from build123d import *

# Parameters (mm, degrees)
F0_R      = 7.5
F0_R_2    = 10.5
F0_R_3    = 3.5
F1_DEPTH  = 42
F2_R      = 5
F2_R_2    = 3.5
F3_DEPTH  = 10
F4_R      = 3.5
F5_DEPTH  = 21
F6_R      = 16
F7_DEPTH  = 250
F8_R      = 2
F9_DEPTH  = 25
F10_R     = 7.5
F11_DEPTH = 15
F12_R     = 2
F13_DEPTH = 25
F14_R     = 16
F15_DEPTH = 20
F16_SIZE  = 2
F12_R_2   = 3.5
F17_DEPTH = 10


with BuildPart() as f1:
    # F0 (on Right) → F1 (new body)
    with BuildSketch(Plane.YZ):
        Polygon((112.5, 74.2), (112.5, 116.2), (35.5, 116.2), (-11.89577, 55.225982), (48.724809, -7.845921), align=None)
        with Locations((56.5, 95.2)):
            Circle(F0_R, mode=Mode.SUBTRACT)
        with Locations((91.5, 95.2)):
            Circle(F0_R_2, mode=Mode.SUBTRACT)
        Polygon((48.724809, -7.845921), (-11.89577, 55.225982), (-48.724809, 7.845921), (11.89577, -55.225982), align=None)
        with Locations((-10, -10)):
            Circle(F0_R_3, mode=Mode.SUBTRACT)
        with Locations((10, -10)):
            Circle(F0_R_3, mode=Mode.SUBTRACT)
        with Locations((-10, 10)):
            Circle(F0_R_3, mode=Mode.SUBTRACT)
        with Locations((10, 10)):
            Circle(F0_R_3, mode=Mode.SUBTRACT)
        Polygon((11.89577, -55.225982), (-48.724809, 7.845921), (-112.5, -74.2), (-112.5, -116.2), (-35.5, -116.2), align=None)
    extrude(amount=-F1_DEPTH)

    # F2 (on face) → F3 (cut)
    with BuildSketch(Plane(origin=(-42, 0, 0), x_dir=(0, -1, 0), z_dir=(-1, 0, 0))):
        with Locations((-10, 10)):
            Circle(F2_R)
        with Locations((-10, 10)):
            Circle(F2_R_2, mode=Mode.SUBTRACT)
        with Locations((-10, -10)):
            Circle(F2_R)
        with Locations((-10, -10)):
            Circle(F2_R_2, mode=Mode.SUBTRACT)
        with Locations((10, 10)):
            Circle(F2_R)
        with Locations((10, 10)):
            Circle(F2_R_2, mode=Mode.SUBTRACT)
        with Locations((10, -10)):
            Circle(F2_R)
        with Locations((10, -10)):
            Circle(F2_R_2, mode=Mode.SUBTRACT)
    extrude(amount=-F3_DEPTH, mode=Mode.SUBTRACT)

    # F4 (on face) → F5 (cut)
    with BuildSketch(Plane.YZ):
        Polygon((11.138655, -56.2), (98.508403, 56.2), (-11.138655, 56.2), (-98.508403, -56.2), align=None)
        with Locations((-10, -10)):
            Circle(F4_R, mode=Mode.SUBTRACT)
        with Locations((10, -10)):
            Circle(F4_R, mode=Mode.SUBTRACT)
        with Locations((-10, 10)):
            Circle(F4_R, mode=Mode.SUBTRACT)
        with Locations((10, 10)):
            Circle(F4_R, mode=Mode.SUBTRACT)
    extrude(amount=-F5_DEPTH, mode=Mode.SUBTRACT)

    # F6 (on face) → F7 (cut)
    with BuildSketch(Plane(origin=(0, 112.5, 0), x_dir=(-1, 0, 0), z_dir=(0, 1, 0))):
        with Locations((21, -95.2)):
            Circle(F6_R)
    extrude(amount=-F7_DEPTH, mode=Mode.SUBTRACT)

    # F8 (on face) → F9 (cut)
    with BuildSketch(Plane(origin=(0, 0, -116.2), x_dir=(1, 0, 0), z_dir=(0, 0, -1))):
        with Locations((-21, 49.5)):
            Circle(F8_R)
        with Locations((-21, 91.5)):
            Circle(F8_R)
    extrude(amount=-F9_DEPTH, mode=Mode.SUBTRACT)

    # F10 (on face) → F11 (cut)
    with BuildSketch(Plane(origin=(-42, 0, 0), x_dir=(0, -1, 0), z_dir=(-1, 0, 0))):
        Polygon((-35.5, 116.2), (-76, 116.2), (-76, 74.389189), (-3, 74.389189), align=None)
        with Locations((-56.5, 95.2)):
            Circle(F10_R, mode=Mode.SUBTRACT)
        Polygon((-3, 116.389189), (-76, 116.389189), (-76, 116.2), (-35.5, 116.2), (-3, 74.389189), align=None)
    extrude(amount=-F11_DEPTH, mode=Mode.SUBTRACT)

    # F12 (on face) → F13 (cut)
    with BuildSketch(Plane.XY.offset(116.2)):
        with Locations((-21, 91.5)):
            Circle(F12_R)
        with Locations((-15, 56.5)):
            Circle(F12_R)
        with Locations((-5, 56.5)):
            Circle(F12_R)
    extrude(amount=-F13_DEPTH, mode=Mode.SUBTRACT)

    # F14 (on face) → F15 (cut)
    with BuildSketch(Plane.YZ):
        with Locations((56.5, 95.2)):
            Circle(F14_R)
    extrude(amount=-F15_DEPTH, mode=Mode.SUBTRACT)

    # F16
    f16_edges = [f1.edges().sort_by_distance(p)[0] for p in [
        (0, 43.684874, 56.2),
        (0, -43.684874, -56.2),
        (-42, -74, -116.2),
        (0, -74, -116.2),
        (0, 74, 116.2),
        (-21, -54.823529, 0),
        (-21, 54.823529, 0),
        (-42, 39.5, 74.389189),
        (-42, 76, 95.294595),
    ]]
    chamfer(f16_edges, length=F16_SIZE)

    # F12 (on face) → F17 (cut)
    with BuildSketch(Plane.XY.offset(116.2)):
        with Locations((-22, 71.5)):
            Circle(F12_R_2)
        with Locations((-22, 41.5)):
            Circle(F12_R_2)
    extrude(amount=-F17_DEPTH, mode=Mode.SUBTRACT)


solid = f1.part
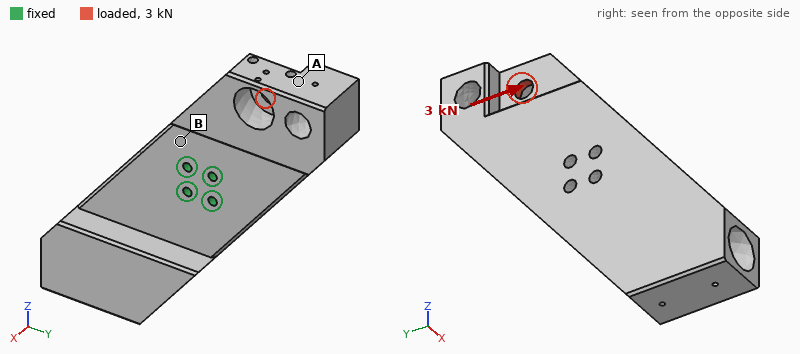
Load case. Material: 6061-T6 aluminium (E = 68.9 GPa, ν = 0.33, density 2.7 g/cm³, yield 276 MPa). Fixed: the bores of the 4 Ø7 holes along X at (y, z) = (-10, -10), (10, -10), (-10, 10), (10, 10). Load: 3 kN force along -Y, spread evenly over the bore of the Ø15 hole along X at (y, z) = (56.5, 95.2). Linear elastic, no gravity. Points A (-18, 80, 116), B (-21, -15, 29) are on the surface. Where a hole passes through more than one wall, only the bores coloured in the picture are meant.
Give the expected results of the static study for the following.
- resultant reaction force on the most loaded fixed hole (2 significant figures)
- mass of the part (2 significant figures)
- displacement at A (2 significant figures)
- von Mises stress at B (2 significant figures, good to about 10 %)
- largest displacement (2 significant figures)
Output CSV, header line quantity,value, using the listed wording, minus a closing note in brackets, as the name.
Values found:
quantity,value
resultant reaction force on the most loaded fixed hole,5.4 kN
mass of the part,1.6 kg
displacement at A,59 µm
von Mises stress at B,8.4 MPa
largest displacement,70 µm
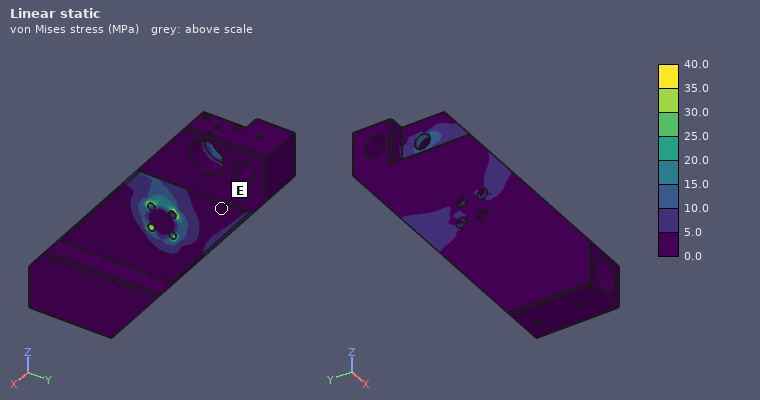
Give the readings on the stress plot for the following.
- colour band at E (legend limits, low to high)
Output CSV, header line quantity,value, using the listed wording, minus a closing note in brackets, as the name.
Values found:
quantity,value
colour band at E,0.0 to 5.0 MPa
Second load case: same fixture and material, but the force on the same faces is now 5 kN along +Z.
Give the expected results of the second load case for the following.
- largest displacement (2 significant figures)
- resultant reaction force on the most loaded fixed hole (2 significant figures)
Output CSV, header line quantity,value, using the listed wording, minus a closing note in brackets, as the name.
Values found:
quantity,value
largest displacement,89 µm
resultant reaction force on the most loaded fixed hole,5.9 kN
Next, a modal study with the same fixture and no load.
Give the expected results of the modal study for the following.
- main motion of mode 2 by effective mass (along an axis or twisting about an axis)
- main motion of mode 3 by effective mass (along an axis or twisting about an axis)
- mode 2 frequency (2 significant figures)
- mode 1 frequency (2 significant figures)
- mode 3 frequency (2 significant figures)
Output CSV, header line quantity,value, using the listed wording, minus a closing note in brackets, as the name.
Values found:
quantity,value
main motion of mode 2 by effective mass,along X
main motion of mode 3 by effective mass,twisting about X
mode 2 frequency,810 Hz
mode 1 frequency,700 Hz
mode 3 frequency,1400 Hz
